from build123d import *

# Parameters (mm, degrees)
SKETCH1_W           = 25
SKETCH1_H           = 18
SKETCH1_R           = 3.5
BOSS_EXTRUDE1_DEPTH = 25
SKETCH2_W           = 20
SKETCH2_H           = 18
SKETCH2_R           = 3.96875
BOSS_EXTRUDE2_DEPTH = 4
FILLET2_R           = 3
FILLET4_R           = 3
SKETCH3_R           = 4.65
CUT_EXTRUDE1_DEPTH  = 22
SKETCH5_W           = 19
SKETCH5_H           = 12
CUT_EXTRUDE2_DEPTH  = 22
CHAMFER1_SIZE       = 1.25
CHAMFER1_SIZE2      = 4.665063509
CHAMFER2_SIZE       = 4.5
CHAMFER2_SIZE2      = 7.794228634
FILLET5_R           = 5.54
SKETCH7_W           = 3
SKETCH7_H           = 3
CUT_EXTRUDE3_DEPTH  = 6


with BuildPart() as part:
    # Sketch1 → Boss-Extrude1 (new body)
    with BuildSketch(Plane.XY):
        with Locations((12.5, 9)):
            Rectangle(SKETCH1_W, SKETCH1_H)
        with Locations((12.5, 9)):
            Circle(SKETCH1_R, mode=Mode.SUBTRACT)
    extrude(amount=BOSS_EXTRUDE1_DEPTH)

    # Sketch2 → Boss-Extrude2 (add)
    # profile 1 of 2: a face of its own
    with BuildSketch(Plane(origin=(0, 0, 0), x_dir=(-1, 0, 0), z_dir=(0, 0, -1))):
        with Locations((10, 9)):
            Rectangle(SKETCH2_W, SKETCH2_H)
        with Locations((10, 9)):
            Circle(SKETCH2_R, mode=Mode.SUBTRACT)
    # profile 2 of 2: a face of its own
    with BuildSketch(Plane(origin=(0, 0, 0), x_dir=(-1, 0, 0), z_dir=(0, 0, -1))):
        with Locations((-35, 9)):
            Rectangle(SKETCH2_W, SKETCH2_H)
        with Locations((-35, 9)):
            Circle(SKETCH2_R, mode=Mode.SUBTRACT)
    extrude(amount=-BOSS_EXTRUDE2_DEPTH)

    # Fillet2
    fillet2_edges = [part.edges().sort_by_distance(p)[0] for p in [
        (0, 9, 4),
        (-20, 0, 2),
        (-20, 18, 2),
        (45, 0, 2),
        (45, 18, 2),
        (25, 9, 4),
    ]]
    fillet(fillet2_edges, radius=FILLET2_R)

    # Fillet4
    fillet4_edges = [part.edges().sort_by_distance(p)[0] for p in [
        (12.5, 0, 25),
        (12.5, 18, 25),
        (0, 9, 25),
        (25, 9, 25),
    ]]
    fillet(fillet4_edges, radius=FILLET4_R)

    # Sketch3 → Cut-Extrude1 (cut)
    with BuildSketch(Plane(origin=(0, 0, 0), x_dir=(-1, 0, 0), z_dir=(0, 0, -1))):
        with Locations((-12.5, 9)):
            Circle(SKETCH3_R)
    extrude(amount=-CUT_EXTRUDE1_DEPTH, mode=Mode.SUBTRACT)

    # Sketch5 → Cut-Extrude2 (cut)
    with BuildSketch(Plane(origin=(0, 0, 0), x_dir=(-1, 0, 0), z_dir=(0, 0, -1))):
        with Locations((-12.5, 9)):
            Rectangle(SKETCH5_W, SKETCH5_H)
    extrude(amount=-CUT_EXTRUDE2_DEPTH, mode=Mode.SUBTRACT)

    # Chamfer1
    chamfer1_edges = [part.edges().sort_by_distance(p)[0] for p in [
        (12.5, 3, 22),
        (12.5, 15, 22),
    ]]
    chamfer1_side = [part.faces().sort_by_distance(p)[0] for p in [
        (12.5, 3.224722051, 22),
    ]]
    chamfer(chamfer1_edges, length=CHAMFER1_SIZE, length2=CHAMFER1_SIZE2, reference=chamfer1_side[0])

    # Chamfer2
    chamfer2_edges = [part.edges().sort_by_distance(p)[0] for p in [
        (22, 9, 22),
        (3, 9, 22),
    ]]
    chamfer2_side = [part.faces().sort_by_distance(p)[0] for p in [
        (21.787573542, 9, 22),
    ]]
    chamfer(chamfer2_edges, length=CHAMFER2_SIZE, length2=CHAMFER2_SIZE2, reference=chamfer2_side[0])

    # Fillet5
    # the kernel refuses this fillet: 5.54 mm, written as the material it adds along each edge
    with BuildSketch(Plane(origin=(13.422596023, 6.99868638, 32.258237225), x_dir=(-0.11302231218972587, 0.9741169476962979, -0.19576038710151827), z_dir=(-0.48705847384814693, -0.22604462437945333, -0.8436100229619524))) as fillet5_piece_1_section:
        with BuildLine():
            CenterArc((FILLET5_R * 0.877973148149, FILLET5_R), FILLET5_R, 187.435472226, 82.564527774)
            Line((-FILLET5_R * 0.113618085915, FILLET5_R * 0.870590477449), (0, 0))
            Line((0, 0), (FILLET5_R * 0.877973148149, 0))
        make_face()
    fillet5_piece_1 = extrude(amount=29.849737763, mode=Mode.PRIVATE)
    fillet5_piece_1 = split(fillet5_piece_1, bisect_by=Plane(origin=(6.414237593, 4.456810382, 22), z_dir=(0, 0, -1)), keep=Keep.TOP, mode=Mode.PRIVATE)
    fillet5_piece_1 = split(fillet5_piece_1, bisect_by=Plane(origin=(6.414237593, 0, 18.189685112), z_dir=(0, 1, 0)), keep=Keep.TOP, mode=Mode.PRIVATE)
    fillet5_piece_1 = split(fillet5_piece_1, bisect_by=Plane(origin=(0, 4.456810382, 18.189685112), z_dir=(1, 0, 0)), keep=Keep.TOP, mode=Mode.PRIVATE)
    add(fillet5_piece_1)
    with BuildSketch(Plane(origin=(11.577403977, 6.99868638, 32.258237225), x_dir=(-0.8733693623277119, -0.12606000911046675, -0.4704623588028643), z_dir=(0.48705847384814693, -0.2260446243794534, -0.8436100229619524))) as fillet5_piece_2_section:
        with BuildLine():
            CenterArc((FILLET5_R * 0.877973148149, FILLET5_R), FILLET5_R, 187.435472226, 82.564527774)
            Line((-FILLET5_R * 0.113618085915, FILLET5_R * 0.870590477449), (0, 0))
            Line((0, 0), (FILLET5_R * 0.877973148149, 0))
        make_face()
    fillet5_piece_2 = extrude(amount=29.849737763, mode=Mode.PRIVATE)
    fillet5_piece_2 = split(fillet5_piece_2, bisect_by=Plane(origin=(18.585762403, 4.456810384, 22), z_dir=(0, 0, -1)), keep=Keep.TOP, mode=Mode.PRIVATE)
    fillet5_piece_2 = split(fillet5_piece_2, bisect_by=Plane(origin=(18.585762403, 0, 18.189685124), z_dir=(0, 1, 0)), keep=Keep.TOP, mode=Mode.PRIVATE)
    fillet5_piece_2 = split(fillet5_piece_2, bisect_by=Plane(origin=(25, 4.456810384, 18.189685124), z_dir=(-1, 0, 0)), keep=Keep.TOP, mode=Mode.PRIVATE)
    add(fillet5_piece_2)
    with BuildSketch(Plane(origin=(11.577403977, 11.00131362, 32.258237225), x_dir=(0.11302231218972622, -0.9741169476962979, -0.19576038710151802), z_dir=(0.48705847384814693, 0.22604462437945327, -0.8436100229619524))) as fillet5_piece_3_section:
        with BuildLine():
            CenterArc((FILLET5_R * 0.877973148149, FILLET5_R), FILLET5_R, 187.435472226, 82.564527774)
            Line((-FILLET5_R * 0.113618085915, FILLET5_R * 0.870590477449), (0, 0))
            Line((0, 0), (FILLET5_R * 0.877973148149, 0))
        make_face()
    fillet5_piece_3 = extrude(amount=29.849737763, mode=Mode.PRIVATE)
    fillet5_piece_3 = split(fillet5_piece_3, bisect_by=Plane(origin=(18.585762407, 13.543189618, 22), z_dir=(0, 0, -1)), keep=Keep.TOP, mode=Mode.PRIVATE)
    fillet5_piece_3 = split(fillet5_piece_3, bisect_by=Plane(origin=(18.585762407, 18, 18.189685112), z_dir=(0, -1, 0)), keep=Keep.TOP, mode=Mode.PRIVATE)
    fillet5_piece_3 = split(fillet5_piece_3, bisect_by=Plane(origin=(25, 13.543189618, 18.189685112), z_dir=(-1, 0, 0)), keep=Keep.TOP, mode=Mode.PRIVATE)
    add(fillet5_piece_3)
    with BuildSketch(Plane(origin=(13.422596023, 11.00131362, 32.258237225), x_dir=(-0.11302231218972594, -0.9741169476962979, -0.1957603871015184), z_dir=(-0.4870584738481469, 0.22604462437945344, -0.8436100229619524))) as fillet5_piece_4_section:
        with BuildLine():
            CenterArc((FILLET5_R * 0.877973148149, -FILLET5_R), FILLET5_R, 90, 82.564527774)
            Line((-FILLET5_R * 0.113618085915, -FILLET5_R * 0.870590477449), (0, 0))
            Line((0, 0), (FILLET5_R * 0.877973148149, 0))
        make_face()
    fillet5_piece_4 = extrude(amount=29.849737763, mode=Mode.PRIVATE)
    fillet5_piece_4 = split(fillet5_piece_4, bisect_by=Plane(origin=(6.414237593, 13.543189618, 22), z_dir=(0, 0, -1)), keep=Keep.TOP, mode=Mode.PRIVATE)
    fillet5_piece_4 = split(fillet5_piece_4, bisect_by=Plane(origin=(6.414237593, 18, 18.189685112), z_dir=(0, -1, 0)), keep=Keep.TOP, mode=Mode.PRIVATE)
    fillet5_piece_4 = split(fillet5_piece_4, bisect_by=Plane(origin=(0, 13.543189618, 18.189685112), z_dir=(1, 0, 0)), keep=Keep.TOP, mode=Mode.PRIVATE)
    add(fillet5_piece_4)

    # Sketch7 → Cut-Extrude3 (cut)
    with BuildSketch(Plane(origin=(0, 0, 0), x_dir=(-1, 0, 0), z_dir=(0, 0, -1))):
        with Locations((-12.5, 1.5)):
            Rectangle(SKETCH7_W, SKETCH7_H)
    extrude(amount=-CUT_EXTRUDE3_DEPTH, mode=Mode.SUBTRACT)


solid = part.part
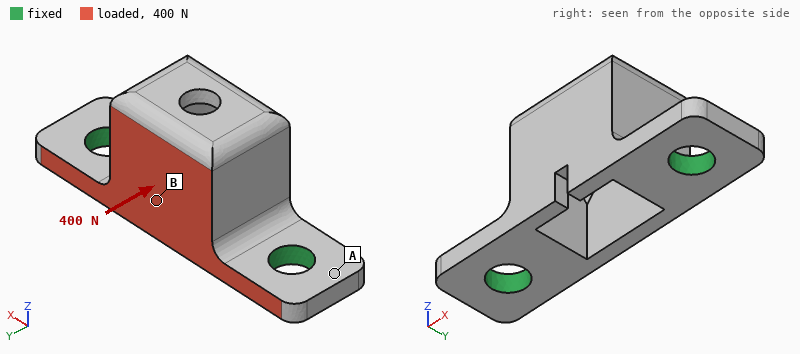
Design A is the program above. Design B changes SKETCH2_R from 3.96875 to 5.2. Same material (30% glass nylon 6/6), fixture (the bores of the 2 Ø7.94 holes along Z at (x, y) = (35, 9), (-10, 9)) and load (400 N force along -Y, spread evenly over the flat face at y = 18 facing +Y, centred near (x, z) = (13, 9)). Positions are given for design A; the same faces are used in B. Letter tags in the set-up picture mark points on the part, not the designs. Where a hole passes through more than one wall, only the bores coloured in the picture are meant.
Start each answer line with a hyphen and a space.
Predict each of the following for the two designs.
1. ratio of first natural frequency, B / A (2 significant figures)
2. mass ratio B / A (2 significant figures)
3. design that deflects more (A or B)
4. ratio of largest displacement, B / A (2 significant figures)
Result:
- 1.2
- 0.97
- A
- 0.73
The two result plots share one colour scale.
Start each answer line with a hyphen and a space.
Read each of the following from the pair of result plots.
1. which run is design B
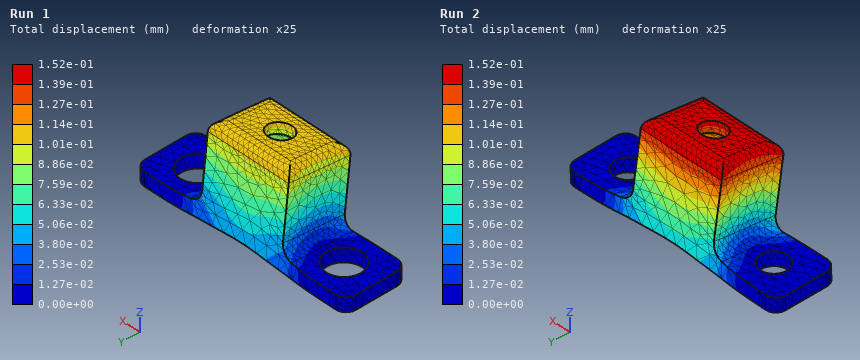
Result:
- Run 1
